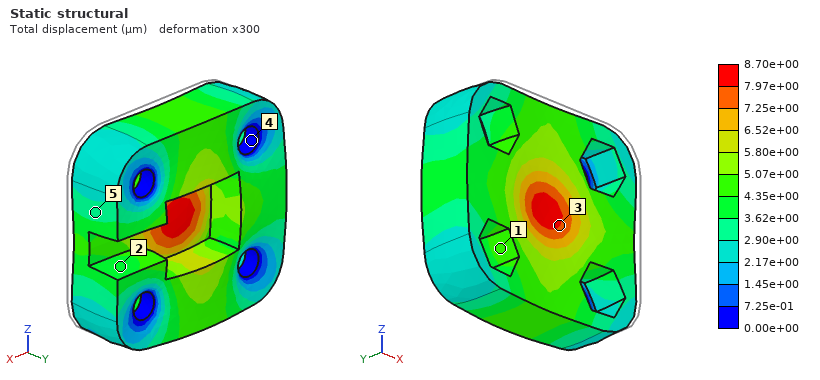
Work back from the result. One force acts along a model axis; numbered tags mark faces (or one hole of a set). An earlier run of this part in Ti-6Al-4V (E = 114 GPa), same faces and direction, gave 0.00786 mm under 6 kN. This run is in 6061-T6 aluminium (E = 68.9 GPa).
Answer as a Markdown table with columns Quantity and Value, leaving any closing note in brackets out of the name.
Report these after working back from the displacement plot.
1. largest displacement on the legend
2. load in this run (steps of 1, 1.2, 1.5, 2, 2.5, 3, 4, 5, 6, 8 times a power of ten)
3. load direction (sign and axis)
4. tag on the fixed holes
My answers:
| Quantity | Value |
|---|---|
| largest displacement on the legend | 8.70e+00 µm |
| load in this run | 4 kN |
| load direction | +Y |
| tag on the fixed holes | 4 |
